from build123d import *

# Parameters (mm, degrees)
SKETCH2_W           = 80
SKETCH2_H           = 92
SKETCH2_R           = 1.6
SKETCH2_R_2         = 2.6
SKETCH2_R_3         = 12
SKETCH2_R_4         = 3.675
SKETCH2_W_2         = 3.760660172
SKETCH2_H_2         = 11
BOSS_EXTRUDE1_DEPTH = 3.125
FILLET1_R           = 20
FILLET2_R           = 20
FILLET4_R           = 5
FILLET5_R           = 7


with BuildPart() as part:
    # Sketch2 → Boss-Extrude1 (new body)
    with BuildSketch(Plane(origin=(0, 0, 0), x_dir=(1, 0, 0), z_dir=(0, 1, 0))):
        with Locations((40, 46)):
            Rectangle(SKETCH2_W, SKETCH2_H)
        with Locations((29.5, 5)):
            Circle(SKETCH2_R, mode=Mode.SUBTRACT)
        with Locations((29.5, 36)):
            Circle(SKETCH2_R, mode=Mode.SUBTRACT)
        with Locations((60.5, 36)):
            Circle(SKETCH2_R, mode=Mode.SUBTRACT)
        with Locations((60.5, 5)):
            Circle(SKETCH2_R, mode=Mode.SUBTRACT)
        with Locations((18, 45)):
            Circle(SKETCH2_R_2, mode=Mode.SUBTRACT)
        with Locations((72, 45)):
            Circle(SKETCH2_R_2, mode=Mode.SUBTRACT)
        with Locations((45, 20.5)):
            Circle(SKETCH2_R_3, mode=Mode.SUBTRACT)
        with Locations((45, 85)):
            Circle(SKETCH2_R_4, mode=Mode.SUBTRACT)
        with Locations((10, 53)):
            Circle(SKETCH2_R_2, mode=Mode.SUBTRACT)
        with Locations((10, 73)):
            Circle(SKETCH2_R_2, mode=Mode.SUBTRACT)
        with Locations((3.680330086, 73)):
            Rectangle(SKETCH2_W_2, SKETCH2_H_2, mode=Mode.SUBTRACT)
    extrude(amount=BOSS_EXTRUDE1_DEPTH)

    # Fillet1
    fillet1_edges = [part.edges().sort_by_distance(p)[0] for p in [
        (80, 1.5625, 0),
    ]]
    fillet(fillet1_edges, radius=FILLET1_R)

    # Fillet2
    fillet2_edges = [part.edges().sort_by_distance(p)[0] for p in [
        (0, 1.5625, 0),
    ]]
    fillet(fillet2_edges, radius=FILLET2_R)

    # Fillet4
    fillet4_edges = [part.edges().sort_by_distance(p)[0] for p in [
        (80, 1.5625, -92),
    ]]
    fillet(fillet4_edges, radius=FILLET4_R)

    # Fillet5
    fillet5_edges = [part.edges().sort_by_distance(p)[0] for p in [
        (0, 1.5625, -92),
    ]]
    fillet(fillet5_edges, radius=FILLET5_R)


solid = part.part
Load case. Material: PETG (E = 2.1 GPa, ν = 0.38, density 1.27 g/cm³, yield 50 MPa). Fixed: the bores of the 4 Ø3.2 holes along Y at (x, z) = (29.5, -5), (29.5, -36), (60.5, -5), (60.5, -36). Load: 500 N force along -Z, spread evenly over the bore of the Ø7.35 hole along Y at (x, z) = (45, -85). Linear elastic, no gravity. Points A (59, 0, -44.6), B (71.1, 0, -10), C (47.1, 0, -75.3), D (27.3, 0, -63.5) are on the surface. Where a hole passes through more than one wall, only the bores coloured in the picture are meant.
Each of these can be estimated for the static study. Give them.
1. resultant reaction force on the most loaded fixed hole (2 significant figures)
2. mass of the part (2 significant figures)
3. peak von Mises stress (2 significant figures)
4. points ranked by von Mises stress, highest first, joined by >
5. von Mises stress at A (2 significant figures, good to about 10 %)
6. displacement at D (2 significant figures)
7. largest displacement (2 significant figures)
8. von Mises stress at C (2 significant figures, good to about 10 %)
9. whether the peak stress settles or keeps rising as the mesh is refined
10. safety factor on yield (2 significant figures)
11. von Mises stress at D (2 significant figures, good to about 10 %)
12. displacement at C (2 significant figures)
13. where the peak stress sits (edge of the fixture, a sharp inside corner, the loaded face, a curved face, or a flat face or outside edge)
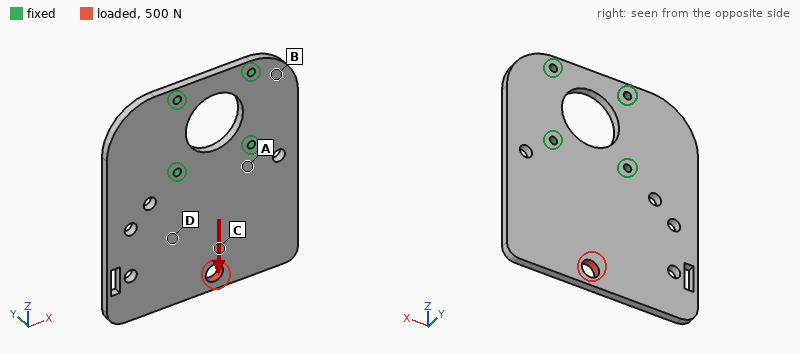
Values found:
230 N
26 g
19 MPa
C > A > D > B
4.6 MPa
0.047 mm
0.17 mm
6.5 MPa
settles
2.6
2.7 MPa
0.090 mm
the loaded face
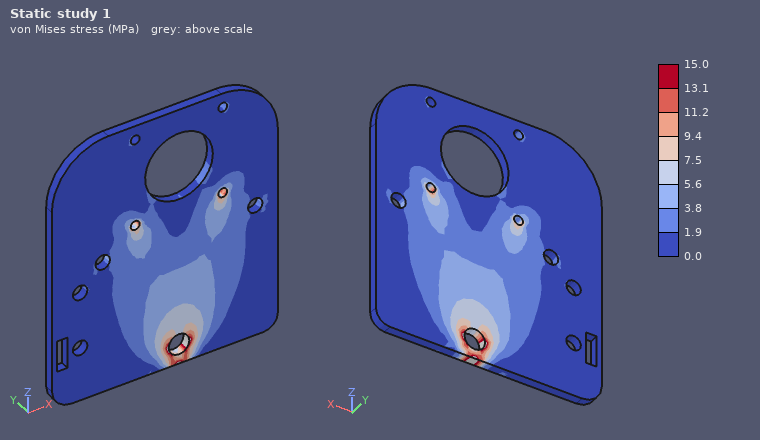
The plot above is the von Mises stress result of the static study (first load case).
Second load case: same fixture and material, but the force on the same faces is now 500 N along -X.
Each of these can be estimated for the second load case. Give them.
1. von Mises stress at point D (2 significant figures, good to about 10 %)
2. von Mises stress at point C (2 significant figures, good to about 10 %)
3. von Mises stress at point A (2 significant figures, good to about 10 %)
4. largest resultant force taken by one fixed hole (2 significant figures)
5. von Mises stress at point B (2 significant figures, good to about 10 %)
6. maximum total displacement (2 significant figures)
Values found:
4.4 MPa
6.6 MPa
8.2 MPa
560 N
2.8 MPa
0.47 mm
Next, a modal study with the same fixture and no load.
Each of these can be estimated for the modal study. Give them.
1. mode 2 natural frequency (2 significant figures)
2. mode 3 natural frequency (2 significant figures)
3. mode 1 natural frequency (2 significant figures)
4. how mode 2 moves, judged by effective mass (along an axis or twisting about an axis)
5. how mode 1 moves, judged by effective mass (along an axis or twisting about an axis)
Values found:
340 Hz
700 Hz
200 Hz
twisting about Z
along Y
